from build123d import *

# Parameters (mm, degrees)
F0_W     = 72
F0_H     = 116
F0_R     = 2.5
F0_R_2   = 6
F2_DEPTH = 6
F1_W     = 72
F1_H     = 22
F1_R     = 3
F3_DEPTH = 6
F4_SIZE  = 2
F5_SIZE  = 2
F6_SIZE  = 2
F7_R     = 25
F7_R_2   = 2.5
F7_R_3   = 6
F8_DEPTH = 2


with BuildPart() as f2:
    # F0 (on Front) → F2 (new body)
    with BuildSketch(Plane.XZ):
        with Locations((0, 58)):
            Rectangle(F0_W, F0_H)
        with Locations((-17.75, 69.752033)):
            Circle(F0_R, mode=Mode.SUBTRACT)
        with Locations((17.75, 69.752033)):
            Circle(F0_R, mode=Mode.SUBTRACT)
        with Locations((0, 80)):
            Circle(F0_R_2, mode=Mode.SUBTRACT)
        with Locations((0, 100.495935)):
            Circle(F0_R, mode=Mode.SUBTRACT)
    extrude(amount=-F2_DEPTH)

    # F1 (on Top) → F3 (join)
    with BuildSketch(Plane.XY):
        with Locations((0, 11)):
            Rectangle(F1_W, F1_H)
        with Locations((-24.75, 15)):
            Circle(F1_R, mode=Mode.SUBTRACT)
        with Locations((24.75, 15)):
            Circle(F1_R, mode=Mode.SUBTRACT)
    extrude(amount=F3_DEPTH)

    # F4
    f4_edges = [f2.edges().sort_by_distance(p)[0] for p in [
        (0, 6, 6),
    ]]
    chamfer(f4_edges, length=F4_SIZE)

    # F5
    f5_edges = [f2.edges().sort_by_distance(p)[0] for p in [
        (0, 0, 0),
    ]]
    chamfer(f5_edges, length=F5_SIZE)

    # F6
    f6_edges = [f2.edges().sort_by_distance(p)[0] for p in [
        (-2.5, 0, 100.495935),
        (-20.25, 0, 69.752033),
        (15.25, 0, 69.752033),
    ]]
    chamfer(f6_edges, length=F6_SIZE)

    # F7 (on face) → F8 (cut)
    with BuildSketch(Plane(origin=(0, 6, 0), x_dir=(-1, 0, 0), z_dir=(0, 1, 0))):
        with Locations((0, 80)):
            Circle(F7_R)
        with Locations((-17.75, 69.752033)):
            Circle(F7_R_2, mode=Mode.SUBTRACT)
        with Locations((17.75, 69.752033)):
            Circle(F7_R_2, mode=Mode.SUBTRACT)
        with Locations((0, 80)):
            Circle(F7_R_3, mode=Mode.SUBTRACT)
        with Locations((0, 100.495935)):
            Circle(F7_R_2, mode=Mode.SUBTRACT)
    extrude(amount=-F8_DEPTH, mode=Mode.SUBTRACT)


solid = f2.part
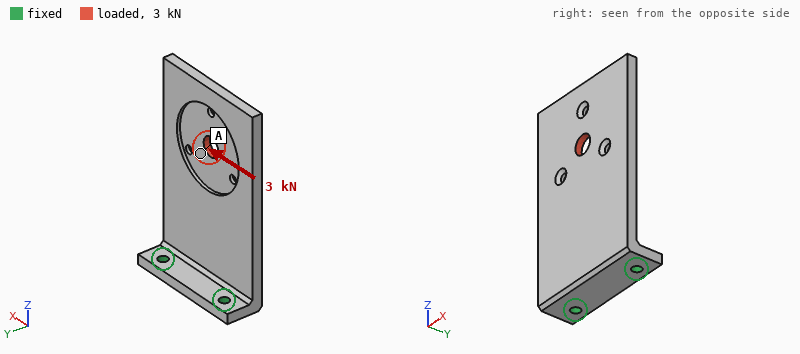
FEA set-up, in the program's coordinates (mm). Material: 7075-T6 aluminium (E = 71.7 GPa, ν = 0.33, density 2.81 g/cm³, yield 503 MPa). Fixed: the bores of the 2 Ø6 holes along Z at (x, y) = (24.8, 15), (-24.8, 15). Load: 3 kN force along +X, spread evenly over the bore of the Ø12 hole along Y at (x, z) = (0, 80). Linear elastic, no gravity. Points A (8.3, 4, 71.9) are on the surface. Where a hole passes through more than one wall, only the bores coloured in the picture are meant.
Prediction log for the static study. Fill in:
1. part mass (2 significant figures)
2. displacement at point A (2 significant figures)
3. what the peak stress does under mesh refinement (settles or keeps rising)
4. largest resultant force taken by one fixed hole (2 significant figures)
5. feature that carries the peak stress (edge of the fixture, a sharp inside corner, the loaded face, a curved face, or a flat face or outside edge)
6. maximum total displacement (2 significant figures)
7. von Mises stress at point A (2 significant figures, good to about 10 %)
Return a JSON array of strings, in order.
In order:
["150 g", "0.20 mm", "keeps rising", "4.7 kN", "edge of the fixture", "0.37 mm", "26 MPa"]
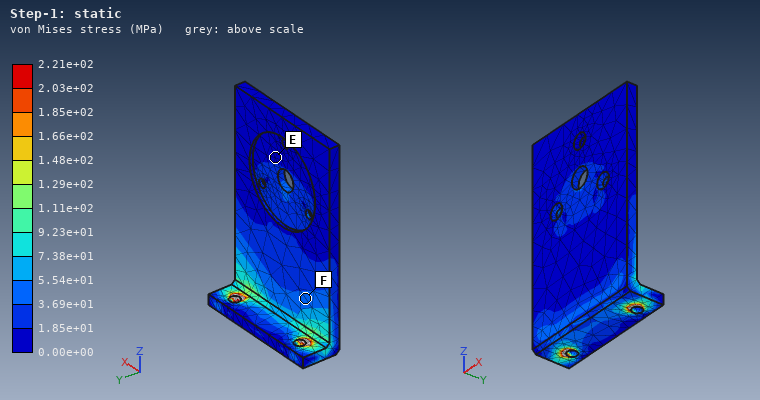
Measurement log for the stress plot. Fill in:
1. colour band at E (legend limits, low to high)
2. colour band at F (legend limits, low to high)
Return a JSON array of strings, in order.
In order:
["0.00e+00 to 1.85e+01 MPa", "3.69e+01 to 5.54e+01 MPa"]
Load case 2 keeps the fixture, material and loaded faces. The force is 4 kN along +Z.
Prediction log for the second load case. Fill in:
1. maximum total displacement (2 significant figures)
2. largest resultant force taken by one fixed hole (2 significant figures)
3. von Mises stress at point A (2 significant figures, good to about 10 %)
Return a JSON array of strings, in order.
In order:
["0.70 mm", "2.0 kN", "25 MPa"]
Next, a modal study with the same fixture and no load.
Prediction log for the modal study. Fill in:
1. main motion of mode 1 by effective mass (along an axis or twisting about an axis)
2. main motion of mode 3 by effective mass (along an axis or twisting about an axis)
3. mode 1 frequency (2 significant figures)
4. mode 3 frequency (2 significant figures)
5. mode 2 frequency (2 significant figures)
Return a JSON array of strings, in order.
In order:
["along Y", "along Y", "350 Hz", "1900 Hz", "1200 Hz"]
